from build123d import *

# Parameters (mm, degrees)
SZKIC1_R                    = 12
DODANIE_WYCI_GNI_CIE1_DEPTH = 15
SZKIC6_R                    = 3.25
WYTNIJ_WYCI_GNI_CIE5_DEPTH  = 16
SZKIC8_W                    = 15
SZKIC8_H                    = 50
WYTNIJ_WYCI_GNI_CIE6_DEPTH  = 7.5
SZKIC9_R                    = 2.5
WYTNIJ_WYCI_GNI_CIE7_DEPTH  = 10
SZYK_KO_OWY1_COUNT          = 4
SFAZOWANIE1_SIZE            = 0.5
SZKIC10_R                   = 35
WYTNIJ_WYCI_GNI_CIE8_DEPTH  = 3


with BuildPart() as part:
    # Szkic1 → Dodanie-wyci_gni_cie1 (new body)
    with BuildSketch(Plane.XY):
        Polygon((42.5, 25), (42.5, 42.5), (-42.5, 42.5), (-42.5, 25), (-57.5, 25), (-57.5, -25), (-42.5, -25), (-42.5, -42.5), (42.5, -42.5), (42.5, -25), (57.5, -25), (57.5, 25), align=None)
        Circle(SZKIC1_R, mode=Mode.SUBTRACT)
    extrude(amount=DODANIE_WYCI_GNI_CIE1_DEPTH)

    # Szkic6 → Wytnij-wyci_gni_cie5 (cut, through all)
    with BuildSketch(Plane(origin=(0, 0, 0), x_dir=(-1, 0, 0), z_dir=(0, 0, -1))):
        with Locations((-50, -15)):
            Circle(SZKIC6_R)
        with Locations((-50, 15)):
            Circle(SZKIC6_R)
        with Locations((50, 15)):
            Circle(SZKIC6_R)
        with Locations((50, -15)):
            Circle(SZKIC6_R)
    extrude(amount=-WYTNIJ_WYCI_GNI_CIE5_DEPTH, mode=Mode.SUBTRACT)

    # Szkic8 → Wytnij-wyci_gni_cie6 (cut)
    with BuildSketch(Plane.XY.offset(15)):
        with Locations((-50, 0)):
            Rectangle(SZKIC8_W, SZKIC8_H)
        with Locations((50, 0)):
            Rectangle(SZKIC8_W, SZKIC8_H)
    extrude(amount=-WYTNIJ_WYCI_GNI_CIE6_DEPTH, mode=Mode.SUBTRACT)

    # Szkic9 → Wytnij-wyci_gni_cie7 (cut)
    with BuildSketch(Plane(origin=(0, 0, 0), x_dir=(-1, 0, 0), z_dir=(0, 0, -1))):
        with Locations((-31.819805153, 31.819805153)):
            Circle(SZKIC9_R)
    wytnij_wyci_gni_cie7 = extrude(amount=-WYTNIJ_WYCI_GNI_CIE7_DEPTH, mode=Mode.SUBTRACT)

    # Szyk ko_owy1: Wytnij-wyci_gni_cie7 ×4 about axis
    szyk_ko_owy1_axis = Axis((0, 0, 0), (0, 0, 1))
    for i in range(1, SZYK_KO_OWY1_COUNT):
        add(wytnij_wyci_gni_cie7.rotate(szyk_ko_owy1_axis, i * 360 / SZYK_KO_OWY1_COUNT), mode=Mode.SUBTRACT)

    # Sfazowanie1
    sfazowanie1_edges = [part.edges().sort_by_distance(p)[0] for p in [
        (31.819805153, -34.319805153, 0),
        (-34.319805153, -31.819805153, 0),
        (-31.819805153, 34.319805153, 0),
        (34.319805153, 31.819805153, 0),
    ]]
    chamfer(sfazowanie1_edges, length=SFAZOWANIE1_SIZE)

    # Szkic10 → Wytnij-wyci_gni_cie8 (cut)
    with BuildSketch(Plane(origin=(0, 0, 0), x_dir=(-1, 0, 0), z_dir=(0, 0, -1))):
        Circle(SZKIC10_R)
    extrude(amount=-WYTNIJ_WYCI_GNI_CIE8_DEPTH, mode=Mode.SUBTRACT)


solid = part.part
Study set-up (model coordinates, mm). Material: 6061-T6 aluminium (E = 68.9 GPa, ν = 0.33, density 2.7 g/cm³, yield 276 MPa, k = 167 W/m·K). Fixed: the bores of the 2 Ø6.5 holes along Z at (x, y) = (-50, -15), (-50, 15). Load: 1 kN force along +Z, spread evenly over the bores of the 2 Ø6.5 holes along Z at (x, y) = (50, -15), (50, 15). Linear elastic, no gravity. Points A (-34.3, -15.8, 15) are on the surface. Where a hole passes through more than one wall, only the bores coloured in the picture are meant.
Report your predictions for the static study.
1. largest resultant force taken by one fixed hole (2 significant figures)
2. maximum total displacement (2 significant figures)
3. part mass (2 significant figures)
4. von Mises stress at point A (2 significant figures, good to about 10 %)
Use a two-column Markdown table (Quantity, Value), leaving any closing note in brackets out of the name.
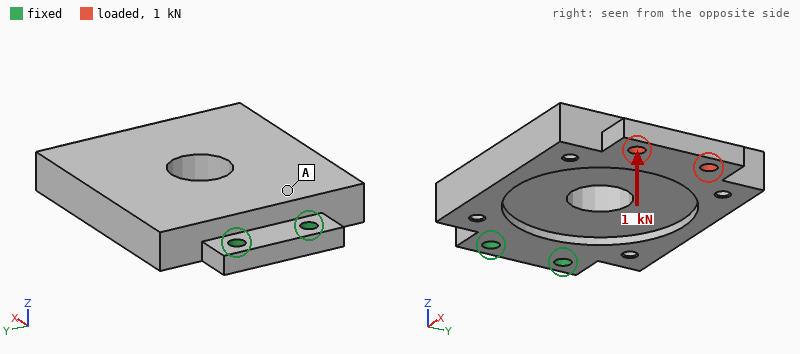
| Quantity | Value |
|---|---|
| largest resultant force taken by one fixed hole | 520 N |
| maximum total displacement | 1.1 mm |
| part mass | 270 g |
| von Mises stress at point A | 32 MPa |
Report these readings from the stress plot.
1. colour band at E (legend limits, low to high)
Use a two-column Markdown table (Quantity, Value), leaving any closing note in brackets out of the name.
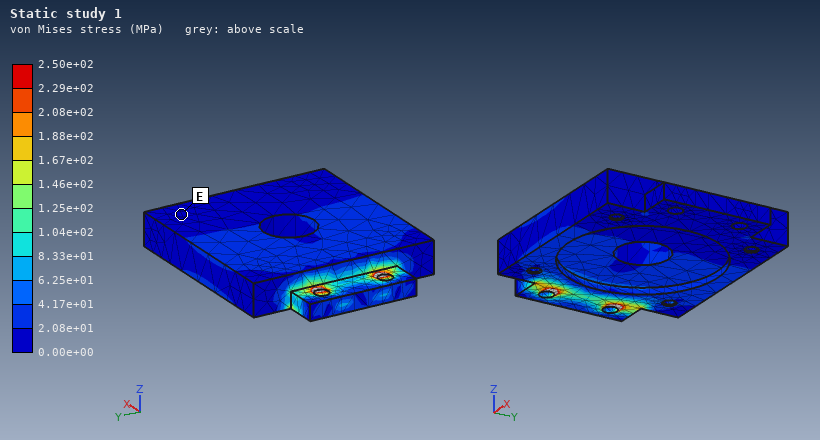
| Quantity | Value |
|---|---|
| colour band at E | 0.00e+00 to 2.08e+01 MPa |
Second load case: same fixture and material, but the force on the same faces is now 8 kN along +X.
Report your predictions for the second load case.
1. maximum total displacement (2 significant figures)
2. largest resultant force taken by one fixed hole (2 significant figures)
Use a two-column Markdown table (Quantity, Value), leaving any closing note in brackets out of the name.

| Quantity | Value |
|---|---|
| maximum total displacement | 0.23 mm |
| largest resultant force taken by one fixed hole | 4.0 kN |
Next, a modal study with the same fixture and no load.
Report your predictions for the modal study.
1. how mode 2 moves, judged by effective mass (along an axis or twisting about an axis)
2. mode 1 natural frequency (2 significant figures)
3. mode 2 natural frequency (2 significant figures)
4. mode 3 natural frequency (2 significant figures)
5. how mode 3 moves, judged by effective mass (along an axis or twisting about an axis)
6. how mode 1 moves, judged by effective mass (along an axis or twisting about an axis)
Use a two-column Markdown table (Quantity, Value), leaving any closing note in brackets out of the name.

| Quantity | Value |
|---|---|
| how mode 2 moves, judged by effective mass | along Y |
| mode 1 natural frequency | 560 Hz |
| mode 2 natural frequency | 1700 Hz |
| mode 3 natural frequency | 2400 Hz |
| how mode 3 moves, judged by effective mass | along Y |
| how mode 1 moves, judged by effective mass | along Z |
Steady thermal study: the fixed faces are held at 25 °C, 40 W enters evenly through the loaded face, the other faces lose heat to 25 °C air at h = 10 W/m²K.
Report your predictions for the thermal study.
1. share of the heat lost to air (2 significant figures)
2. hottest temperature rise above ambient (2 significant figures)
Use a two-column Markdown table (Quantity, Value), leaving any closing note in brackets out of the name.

| Quantity | Value |
|---|---|
| share of the heat lost to air | 10 % |
| hottest temperature rise above ambient | 37 K |
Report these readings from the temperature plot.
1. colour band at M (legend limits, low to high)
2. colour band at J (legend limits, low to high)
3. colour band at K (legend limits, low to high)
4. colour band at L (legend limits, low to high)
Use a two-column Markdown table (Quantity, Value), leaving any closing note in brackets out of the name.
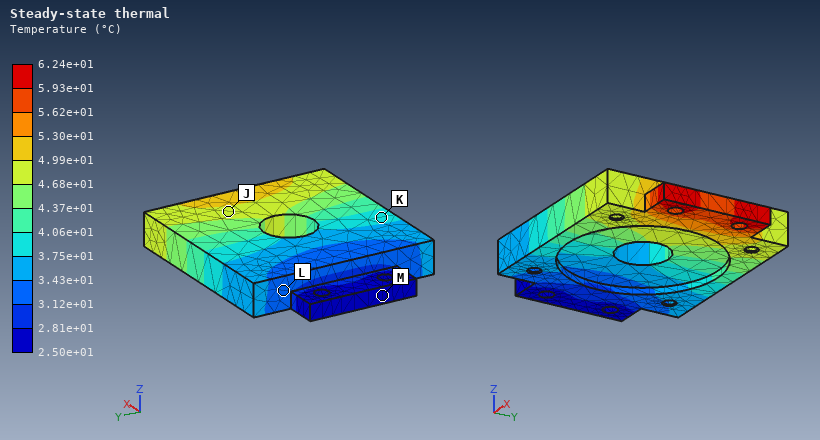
| Quantity | Value |
|---|---|
| colour band at M | 2.50e+01 to 2.81e+01 °C |
| colour band at J | 4.68e+01 to 4.99e+01 °C |
| colour band at K | 3.75e+01 to 4.06e+01 °C |
| colour band at L | 3.12e+01 to 3.43e+01 °C |
